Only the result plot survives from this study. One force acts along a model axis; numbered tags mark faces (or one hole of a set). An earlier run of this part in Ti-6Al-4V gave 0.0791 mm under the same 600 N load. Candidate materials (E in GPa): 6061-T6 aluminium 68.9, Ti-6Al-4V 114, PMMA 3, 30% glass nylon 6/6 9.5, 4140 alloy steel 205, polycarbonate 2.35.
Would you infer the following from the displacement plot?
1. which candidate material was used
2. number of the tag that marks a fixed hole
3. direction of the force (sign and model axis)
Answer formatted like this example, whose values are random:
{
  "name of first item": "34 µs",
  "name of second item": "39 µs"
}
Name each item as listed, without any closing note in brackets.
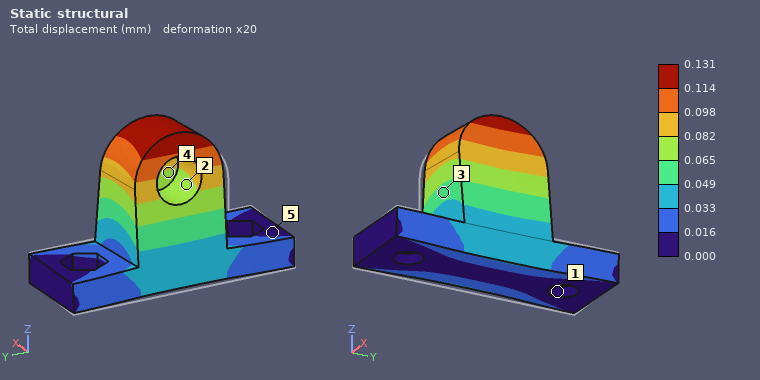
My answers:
{
  "which candidate material was used": "6061-T6 aluminium",
  "number of the tag that marks a fixed hole": "1",
  "direction of the force": "+X"
}
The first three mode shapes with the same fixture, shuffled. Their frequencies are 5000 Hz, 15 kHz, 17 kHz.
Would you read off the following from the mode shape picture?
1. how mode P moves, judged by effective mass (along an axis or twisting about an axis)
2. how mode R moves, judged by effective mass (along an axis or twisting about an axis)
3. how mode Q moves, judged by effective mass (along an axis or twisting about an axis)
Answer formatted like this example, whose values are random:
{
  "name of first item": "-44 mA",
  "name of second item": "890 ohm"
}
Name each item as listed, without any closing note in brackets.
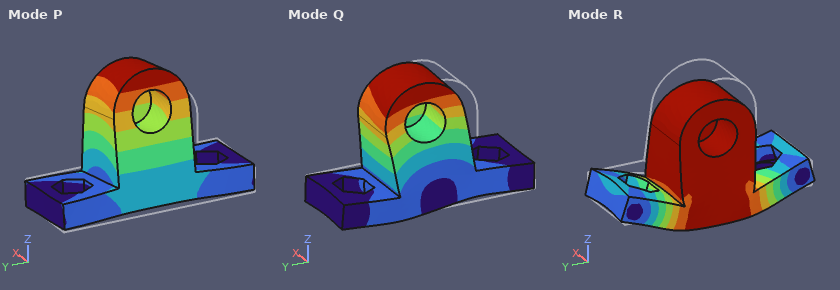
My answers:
{
  "how mode P moves, judged by effective mass": "along X",
  "how mode R moves, judged by effective mass": "along Z",
  "how mode Q moves, judged by effective mass": "along Y"
}
